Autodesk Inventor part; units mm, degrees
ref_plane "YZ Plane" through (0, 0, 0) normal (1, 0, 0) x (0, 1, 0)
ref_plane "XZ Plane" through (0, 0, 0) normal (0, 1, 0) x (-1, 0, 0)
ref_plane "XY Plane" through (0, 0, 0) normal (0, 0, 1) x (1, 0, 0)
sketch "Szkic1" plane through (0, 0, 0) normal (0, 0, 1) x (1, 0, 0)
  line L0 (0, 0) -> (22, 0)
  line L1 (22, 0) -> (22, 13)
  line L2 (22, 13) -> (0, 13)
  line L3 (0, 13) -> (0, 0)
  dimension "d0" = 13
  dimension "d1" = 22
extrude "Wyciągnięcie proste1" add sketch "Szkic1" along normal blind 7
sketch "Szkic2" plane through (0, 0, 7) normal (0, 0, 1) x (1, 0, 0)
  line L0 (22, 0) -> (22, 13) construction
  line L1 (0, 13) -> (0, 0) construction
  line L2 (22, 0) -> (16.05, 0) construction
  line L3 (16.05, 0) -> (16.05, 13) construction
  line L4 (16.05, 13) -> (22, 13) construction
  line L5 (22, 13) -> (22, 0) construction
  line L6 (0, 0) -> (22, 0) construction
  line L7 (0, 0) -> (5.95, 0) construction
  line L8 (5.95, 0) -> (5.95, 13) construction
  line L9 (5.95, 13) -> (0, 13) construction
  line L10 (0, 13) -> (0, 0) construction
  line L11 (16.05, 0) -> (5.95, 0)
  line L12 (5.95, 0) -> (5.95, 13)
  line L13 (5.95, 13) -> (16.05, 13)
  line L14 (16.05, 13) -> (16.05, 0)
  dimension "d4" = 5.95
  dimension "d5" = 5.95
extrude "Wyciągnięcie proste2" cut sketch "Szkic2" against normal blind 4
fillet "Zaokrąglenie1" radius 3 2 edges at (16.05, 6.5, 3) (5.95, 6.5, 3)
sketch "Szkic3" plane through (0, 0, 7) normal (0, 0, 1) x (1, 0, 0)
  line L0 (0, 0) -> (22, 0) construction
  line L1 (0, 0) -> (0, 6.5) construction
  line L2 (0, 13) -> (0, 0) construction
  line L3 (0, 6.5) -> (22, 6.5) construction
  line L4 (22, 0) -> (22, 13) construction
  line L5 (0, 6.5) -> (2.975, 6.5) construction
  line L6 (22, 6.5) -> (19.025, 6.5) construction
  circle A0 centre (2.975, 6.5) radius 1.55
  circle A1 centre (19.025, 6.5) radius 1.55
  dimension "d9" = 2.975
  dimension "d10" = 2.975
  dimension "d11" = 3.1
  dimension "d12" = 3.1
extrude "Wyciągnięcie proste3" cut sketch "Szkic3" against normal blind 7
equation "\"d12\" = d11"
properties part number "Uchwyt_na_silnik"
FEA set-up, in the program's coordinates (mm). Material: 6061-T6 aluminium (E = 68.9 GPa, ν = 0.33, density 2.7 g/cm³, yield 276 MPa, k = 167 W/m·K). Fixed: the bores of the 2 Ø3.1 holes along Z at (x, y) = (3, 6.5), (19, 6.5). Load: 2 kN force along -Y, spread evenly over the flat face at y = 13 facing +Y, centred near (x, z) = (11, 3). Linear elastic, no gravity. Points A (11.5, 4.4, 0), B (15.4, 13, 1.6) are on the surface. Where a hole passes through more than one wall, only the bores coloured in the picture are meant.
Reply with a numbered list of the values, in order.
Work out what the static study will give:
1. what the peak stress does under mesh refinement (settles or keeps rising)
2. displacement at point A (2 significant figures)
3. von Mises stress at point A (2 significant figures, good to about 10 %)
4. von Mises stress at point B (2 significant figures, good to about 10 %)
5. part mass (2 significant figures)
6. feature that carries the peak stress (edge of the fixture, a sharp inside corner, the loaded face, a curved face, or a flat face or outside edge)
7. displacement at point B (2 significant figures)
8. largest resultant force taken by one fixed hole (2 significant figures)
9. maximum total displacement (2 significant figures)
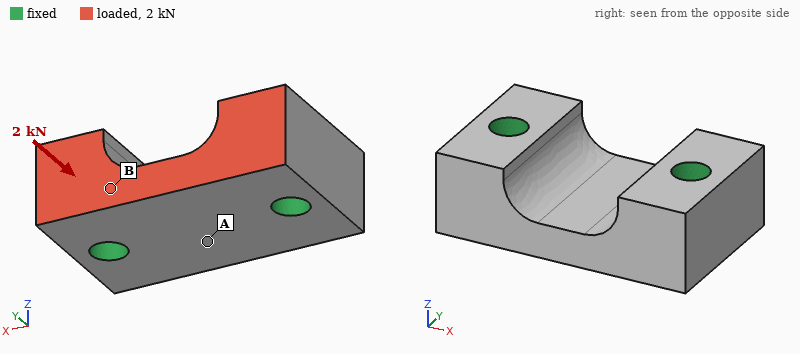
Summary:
1. keeps rising
2. 1.9 µm
3. 6.2 MPa
4. 15 MPa
5. 3.8 g
6. edge of the fixture
7. 2.4 µm
8. 1.0 kN
9. 3.4 µm
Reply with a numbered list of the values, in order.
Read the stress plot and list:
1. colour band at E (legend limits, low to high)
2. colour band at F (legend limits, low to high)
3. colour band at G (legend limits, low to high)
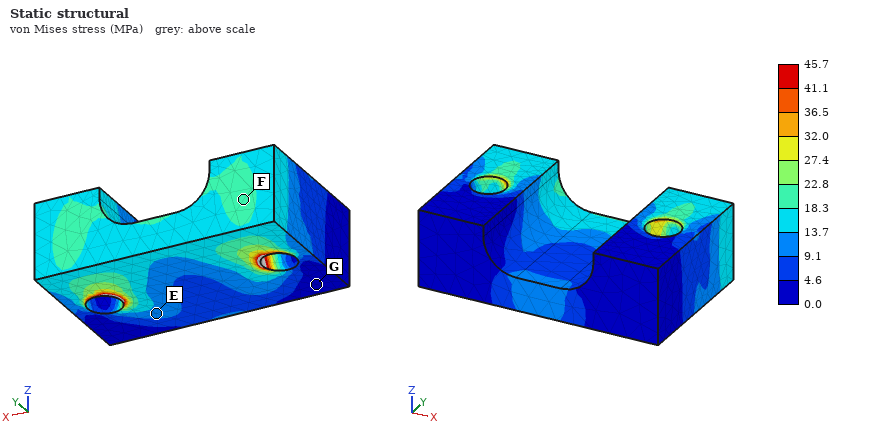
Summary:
1. 9.1 to 13.7 MPa
2. 18.3 to 22.8 MPa
3. 0.0 to 4.6 MPa
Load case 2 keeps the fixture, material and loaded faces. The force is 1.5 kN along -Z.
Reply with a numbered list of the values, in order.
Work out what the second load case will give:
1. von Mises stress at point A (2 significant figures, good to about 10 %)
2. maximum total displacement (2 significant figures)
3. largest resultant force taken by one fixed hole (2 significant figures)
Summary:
1. 13 MPa
2. 14 µm
3. 750 N
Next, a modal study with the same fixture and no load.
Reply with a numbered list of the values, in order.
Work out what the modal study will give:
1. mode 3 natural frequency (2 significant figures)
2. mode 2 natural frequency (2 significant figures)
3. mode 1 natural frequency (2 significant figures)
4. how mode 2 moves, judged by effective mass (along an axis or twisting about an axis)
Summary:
1. 87 kHz
2. 74 kHz
3. 69 kHz
4. along Z
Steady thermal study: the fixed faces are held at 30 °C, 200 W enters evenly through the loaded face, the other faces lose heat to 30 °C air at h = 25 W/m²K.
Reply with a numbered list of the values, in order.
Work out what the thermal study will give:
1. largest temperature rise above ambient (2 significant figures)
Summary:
1. 73 K
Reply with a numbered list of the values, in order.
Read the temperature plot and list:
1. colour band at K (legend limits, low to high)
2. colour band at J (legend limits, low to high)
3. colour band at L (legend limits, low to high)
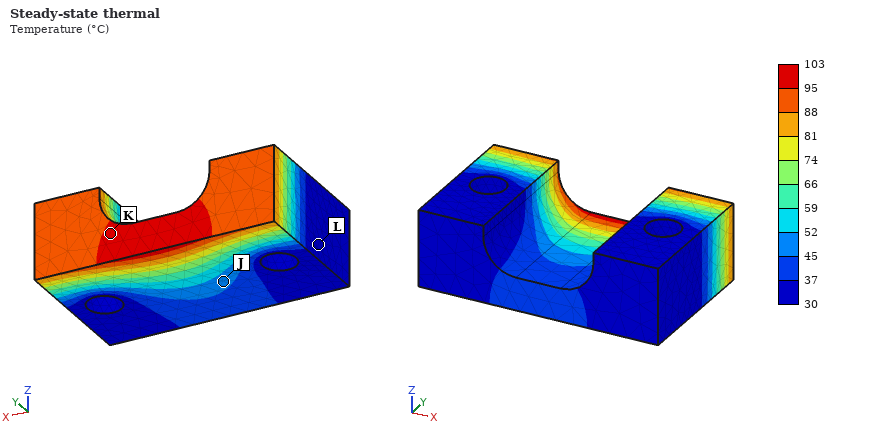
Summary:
1. 95 to 103 °C
2. 45 to 52 °C
3. 30 to 37 °C
